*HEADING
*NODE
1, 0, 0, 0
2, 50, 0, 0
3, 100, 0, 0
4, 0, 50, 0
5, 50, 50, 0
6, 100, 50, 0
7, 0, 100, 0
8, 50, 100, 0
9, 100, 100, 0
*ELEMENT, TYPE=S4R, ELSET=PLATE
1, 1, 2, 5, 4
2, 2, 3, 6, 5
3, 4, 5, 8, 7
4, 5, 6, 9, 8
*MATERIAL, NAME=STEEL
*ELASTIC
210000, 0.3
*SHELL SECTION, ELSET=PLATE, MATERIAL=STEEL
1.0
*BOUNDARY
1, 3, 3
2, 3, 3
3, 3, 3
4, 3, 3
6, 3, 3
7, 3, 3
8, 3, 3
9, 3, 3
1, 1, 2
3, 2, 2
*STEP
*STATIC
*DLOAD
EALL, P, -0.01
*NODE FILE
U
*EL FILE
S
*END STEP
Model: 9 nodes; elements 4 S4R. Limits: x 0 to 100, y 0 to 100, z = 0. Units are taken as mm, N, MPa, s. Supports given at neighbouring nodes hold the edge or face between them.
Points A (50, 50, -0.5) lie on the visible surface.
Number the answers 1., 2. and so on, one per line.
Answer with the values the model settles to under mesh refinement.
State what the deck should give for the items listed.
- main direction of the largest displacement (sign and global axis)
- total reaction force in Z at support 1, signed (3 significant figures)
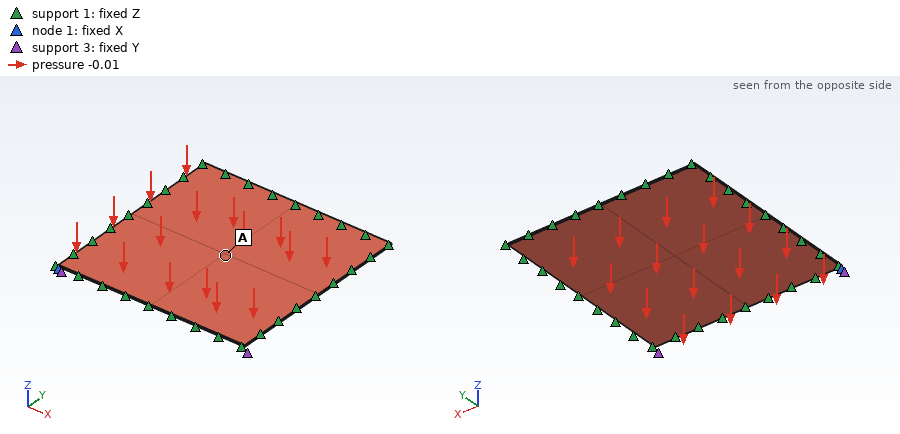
1. -Z
2. 100 N
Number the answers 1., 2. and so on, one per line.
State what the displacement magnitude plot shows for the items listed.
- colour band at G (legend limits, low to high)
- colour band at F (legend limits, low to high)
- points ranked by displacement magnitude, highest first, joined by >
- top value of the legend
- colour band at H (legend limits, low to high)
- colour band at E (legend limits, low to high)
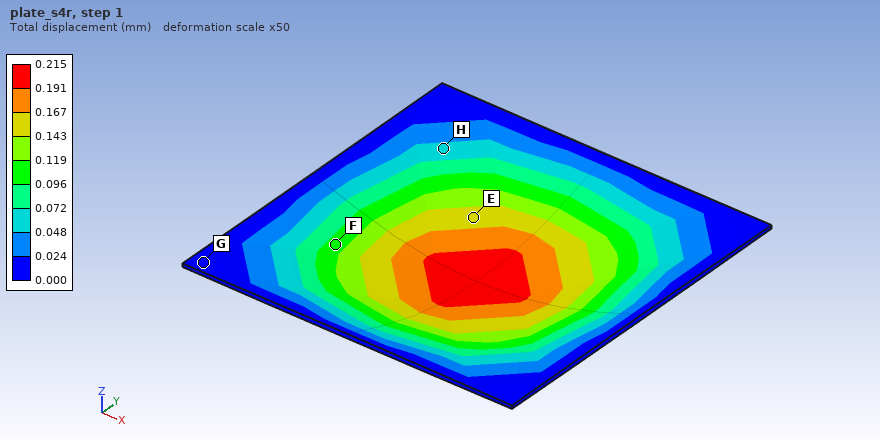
1. 0.000 to 0.024 mm
2. 0.096 to 0.119 mm
3. E > F > H > G
4. 0.215 mm
5. 0.048 to 0.072 mm
6. 0.143 to 0.167 mm
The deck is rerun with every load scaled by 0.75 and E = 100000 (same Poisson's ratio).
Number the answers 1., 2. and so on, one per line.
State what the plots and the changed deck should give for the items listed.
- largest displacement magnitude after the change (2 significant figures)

1. 0.34 mm
